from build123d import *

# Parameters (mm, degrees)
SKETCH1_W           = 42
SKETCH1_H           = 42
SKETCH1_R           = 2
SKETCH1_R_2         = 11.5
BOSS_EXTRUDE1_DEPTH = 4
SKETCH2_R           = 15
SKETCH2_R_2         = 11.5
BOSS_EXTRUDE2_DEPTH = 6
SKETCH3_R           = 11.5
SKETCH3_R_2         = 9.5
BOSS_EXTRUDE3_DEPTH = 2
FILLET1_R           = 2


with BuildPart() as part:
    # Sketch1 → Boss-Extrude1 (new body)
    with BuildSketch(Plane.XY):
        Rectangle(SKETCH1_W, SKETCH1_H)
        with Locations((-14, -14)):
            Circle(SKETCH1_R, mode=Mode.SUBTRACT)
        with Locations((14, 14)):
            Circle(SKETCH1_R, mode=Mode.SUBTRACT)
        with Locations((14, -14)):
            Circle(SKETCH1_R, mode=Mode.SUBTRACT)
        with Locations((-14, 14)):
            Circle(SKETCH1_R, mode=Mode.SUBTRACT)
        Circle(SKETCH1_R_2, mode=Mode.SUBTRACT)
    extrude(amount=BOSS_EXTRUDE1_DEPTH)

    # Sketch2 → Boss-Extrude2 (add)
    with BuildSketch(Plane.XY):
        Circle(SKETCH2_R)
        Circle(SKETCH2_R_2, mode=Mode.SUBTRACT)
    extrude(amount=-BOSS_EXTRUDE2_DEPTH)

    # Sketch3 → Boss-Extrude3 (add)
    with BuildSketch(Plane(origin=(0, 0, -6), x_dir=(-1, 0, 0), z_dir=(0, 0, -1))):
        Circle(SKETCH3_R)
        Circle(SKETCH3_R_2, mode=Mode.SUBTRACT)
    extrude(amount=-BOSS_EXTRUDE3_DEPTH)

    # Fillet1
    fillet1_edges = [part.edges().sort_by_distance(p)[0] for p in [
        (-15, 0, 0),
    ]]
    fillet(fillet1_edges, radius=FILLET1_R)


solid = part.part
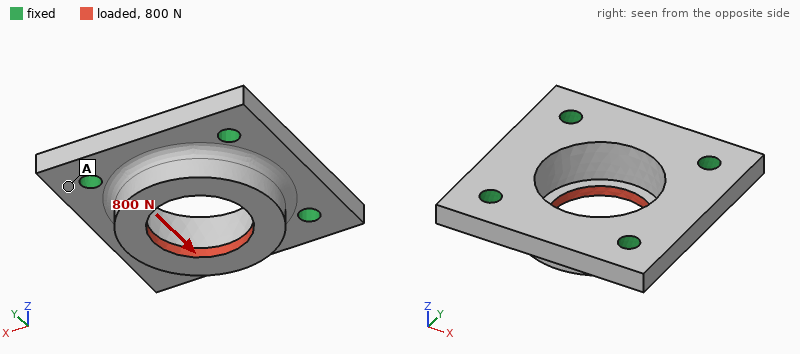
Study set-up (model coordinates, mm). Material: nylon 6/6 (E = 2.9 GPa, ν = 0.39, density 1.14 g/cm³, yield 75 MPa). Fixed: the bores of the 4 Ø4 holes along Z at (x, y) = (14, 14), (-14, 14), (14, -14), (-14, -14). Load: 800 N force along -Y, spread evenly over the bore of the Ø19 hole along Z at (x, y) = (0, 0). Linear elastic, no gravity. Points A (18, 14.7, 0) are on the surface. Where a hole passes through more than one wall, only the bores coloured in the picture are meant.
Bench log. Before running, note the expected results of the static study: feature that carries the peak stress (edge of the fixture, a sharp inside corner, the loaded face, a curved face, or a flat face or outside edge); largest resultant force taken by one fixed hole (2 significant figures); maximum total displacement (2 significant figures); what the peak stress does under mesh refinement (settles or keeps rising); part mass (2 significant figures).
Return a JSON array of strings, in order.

["edge of the fixture", "220 N", "0.11 mm", "keeps rising", "8.3 g"]
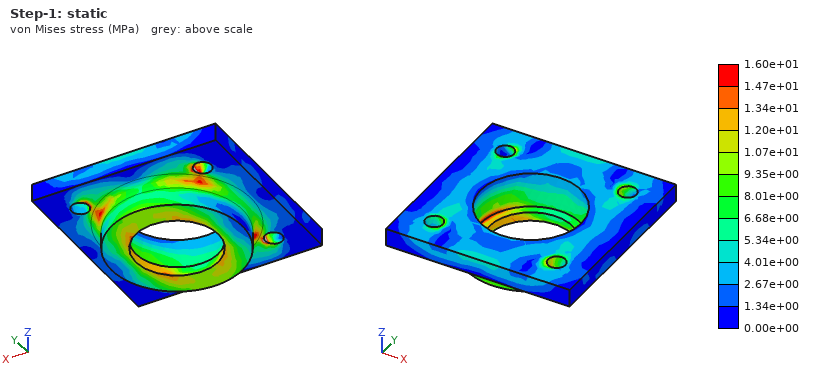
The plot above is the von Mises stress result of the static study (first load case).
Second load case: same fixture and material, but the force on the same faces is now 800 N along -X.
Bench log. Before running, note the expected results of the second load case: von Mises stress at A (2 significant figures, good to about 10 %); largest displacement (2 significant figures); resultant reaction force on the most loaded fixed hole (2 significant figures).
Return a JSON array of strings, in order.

["1.7 MPa", "0.11 mm", "220 N"]
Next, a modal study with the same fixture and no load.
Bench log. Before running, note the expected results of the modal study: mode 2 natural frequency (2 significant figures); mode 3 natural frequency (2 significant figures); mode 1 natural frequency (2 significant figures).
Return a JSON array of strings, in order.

["8900 Hz", "9100 Hz", "8300 Hz"]
